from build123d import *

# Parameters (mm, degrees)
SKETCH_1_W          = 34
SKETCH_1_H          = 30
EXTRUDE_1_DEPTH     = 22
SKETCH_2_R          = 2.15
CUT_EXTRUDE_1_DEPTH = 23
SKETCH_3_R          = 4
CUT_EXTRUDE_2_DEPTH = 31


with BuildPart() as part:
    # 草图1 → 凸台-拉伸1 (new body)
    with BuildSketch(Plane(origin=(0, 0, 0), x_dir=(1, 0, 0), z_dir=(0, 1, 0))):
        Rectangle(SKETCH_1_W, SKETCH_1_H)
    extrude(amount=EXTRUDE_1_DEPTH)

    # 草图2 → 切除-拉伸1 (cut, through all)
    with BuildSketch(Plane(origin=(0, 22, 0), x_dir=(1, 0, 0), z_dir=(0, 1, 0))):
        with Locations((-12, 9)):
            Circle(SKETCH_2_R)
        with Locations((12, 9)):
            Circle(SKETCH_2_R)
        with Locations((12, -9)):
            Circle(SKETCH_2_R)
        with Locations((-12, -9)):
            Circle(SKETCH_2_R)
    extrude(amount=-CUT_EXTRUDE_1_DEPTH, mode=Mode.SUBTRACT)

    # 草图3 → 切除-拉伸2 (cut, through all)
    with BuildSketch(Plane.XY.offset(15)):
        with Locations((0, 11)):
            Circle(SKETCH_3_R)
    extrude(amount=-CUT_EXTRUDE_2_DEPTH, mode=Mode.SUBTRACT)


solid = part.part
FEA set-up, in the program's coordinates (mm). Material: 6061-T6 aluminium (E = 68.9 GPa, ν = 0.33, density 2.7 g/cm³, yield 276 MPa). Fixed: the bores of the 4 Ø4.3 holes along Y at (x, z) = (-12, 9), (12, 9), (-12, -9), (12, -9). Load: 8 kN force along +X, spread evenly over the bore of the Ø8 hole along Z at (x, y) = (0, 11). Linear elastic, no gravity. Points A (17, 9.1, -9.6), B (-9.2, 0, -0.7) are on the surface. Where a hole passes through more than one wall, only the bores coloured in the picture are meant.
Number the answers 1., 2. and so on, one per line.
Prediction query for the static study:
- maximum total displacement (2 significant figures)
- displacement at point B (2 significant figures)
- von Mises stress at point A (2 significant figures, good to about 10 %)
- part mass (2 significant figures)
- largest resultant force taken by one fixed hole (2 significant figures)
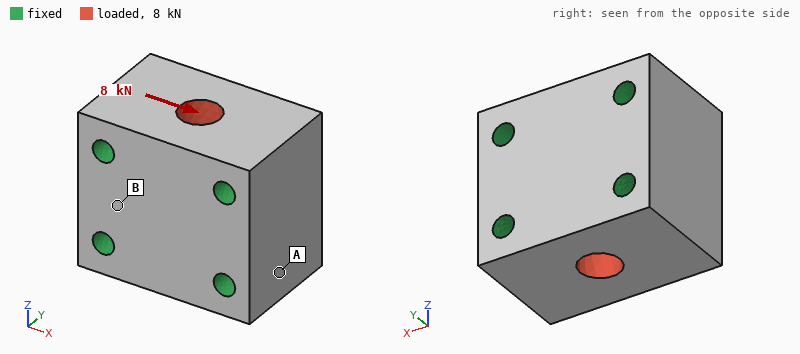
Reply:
1. 1.6 µm
2. 0.70 µm
3. 3.6 MPa
4. 53 g
5. 2.0 kN
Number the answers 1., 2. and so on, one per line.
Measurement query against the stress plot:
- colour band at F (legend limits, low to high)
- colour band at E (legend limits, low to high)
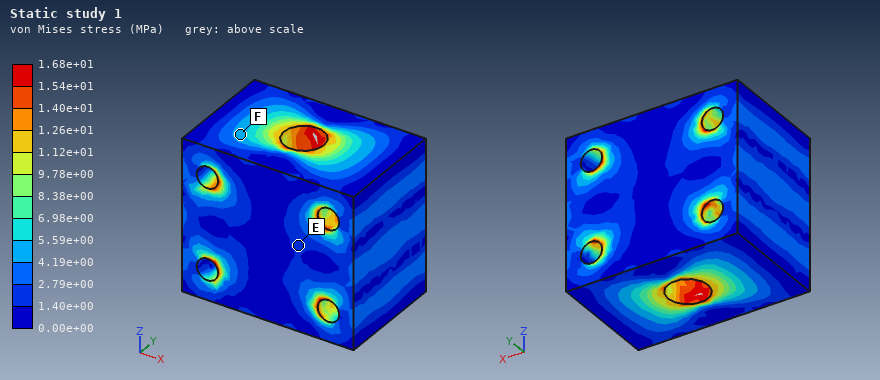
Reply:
1. 4.19e+00 to 5.59e+00 MPa
2. 1.40e+00 to 2.79e+00 MPa
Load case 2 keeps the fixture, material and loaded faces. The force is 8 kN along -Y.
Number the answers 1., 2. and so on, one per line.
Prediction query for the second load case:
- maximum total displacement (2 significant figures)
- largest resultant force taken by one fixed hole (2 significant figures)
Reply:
1. 3.3 µm
2. 2.0 kN
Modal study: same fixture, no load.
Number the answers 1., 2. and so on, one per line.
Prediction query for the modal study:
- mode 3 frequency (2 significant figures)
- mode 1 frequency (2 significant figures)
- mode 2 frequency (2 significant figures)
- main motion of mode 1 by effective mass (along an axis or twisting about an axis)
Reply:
1. 67 kHz
2. 61 kHz
3. 65 kHz
4. along Y
